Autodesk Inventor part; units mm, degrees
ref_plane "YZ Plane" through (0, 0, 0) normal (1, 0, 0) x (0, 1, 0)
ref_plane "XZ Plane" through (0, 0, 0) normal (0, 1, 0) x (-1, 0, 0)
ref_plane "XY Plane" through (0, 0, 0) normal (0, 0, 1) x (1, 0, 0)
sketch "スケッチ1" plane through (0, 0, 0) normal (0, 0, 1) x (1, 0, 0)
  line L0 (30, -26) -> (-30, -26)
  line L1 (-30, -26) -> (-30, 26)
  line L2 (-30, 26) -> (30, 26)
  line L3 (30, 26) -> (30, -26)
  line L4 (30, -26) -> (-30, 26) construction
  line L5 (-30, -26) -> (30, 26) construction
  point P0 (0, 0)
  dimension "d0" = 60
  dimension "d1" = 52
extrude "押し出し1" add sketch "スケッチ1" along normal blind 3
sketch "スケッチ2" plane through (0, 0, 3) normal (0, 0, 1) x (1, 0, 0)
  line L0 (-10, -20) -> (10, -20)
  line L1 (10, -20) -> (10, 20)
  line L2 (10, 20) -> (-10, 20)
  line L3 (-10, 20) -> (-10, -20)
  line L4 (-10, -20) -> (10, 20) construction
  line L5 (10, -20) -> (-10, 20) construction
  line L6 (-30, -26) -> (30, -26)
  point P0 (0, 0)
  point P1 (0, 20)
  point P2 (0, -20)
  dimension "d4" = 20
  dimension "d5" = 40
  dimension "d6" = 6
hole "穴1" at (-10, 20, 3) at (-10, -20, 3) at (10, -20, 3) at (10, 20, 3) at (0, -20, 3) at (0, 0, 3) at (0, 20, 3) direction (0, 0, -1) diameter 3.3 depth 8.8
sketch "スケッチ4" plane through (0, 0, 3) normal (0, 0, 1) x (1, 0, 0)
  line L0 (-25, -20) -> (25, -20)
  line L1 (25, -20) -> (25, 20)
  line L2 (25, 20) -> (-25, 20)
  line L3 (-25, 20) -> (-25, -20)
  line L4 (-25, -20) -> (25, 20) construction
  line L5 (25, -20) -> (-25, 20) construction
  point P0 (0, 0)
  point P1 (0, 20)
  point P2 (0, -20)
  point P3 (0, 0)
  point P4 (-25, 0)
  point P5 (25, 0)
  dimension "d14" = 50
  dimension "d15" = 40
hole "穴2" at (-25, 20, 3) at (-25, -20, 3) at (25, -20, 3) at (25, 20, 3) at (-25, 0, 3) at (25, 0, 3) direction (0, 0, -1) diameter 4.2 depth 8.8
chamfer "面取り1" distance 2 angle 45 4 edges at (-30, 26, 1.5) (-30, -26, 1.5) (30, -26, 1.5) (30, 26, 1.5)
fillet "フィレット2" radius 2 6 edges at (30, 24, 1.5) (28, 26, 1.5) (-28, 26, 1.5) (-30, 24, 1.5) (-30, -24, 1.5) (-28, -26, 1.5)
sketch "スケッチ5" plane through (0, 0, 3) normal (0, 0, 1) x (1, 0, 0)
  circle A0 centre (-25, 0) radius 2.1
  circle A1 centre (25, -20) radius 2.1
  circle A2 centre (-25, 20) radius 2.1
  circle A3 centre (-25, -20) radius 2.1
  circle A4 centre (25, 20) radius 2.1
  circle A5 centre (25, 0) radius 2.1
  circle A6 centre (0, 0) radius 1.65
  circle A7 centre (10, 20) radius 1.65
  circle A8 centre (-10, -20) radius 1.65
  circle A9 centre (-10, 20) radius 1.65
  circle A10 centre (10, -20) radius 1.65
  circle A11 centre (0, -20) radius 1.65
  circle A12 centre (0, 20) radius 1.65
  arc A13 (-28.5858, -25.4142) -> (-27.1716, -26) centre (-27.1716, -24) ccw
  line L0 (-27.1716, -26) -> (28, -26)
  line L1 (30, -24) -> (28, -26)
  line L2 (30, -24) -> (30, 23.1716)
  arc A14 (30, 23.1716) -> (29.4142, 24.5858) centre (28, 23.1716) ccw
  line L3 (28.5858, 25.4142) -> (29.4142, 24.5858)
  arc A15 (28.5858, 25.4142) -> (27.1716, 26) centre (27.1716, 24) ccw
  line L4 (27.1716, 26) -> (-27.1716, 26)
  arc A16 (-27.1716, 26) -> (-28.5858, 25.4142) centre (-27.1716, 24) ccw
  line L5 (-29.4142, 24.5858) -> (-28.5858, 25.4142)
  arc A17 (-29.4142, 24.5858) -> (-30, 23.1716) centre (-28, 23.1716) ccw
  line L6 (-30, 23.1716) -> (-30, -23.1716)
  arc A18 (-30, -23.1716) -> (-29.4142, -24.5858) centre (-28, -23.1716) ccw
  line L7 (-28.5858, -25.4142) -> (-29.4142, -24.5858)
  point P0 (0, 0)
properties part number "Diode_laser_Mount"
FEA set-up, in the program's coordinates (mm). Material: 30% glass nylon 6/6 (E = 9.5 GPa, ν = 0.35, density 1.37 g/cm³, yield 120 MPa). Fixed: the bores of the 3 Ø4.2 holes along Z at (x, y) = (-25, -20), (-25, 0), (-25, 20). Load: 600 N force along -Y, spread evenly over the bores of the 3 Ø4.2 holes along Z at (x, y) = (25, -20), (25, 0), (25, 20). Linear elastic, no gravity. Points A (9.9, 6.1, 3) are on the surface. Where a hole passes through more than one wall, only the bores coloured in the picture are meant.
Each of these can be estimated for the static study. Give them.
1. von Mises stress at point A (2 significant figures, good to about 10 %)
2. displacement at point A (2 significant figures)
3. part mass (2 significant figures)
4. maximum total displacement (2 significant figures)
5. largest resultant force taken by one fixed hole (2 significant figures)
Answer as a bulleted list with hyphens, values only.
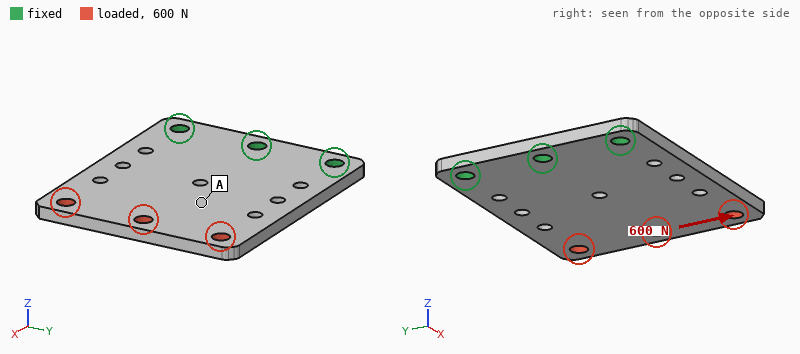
- 9.8 MPa
- 0.097 mm
- 12 g
- 0.19 mm
- 740 N
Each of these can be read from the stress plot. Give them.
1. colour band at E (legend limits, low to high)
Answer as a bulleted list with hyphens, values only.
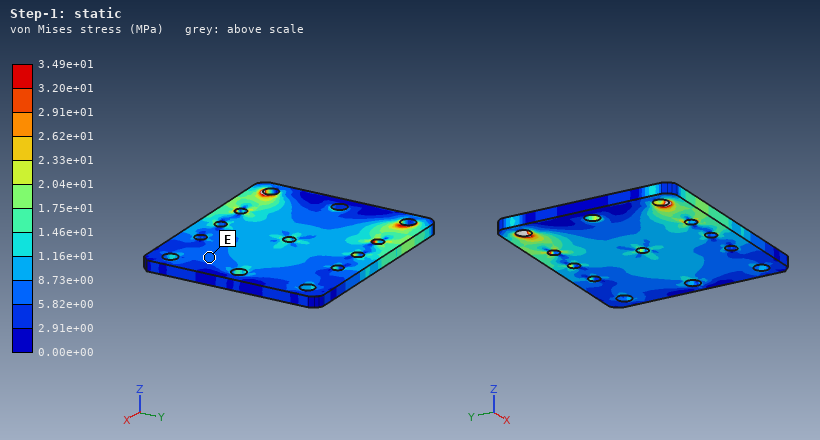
- 5.82e+00 to 8.73e+00 MPa
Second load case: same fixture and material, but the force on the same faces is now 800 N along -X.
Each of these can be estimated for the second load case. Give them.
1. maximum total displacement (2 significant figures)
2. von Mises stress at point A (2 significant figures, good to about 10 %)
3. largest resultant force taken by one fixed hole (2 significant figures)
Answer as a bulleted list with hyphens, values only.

- 39 µm
- 4.8 MPa
- 290 N
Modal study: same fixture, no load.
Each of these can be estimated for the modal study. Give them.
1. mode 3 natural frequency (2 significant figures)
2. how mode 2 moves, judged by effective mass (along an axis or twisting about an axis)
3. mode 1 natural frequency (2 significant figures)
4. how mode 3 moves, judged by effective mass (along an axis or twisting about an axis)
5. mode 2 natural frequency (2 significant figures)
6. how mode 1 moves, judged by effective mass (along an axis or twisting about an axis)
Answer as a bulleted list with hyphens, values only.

- 2700 Hz
- twisting about X
- 440 Hz
- along Z
- 1100 Hz
- along Z
